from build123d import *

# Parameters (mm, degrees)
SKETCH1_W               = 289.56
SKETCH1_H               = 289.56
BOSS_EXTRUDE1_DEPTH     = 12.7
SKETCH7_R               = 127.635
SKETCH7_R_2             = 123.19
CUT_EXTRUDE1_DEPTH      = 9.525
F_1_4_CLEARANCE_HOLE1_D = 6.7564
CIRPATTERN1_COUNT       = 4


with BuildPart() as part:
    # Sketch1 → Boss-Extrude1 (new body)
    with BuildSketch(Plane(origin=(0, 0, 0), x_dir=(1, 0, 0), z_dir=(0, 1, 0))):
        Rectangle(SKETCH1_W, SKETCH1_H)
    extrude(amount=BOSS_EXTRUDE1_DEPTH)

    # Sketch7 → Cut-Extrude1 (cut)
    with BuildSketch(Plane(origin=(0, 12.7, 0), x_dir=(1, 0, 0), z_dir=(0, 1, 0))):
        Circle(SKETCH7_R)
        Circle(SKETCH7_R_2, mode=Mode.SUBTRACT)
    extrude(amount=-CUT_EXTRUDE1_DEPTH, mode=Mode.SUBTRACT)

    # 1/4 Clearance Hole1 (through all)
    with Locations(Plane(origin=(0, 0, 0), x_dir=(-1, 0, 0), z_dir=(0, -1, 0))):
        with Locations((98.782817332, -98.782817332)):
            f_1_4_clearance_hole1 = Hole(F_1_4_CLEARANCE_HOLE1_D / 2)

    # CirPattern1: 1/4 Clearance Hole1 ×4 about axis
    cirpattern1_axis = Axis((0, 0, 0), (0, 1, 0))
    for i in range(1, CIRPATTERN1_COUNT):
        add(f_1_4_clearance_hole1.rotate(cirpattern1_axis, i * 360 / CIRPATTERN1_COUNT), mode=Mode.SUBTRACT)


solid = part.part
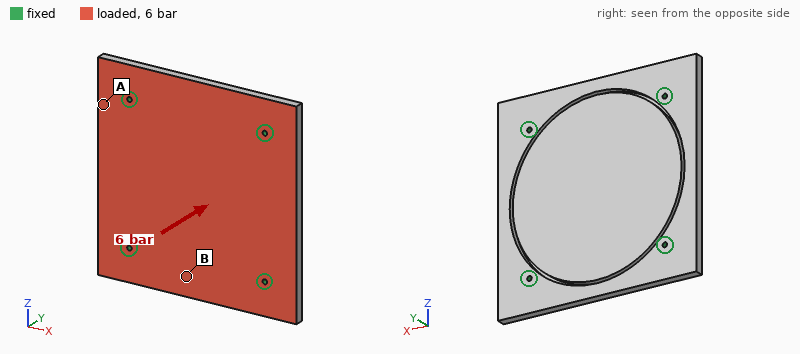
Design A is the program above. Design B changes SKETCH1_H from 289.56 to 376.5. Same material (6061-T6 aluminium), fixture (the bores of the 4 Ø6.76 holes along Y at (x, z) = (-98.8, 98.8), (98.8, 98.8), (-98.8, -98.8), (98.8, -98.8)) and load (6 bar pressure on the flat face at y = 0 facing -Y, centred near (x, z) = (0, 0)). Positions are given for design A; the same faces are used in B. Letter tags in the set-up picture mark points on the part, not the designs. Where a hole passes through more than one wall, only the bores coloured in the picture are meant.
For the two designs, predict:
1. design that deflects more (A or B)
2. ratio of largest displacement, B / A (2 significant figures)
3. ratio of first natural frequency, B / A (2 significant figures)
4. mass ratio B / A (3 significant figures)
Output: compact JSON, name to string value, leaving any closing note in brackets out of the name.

{"design that deflects more": "B", "ratio of largest displacement, B / A": "1.4", "ratio of first natural frequency, B / A": "0.83", "mass ratio B / A": "1.31"}
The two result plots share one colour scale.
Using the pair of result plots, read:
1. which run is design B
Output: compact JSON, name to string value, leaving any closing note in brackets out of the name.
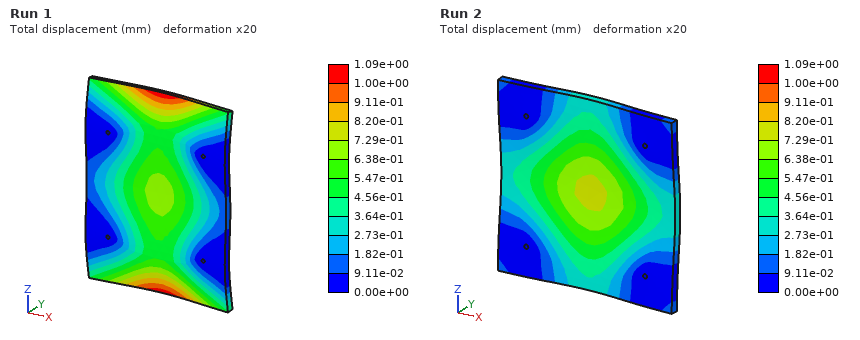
{"which run is design B": "Run 1"}
